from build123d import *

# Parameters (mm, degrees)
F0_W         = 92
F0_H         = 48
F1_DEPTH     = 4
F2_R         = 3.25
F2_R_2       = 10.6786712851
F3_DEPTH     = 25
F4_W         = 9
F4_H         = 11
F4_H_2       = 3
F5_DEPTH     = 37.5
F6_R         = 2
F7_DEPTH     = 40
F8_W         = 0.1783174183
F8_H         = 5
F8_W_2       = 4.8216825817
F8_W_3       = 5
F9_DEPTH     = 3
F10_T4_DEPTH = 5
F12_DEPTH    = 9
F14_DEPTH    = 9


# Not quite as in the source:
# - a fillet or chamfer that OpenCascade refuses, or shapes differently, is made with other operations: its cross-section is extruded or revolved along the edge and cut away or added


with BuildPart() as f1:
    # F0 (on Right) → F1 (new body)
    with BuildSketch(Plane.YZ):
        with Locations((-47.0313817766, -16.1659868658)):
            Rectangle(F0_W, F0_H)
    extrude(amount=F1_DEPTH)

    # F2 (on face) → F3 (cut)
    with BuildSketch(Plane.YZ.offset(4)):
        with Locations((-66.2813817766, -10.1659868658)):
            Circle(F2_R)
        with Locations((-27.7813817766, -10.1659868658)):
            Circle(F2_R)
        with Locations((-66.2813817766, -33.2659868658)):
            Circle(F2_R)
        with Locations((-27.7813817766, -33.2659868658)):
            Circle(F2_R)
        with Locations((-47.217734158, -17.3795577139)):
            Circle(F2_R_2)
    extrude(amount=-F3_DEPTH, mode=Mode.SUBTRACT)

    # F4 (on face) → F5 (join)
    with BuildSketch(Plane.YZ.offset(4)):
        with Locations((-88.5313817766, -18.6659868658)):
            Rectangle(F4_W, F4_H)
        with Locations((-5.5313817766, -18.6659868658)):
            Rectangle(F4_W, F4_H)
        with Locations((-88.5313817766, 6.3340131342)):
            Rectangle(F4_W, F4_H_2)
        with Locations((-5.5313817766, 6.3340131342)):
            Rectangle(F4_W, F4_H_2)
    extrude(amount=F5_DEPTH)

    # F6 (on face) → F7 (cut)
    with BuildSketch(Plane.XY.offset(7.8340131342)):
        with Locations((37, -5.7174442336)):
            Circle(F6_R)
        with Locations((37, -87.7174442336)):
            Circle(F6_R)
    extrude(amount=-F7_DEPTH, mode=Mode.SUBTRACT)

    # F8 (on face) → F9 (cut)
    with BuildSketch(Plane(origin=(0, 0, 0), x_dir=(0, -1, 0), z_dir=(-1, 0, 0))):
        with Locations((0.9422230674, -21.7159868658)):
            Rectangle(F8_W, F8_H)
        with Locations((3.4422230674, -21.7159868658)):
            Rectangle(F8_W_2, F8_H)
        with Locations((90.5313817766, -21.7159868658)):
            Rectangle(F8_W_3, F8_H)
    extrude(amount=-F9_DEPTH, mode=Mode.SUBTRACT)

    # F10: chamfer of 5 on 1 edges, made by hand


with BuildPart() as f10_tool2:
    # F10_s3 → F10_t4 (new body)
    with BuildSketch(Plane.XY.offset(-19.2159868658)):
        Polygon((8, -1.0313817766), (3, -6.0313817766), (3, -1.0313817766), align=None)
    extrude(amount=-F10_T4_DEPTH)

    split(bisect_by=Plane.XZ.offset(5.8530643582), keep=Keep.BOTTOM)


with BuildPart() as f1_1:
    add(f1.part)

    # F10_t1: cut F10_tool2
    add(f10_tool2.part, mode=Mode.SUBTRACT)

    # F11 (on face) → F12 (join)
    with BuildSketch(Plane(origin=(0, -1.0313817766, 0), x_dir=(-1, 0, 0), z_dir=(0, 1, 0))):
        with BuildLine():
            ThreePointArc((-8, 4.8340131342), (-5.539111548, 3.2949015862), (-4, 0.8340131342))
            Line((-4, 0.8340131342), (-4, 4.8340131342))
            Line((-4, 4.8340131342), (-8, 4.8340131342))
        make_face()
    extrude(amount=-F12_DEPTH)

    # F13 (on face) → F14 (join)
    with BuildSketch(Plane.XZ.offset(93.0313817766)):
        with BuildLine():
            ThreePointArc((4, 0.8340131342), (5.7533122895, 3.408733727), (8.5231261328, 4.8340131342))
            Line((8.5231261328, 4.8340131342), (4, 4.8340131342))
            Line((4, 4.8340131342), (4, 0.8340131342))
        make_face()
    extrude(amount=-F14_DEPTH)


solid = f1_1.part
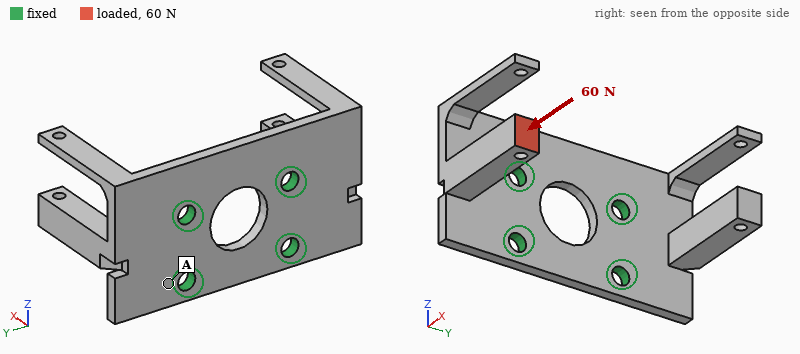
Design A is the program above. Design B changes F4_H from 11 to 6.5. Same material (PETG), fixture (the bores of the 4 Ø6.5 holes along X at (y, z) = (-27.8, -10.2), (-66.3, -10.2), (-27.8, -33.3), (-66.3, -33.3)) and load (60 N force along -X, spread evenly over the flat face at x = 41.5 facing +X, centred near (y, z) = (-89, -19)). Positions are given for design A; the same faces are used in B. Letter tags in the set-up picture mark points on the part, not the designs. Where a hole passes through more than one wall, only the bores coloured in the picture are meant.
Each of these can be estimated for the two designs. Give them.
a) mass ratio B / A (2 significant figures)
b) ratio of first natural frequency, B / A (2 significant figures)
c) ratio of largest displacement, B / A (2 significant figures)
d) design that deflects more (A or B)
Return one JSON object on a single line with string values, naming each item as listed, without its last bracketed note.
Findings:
{"mass ratio B / A": "0.88", "ratio of first natural frequency, B / A": "1.1", "ratio of largest displacement, B / A": "1.1", "design that deflects more": "B"}
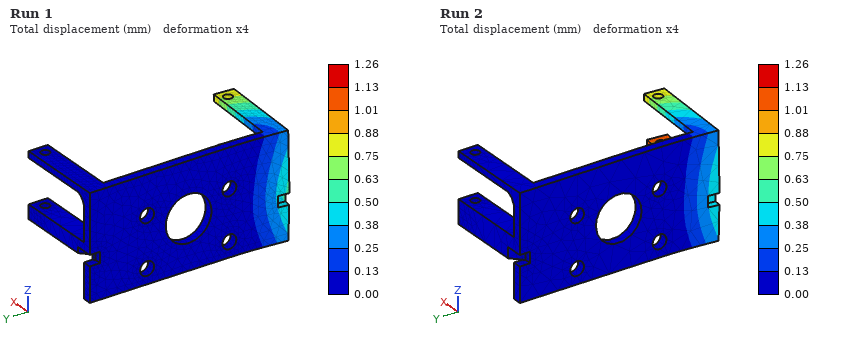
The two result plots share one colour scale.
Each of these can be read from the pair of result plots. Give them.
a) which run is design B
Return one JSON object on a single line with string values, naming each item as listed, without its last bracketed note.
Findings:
{"which run is design B": "Run 1"}
